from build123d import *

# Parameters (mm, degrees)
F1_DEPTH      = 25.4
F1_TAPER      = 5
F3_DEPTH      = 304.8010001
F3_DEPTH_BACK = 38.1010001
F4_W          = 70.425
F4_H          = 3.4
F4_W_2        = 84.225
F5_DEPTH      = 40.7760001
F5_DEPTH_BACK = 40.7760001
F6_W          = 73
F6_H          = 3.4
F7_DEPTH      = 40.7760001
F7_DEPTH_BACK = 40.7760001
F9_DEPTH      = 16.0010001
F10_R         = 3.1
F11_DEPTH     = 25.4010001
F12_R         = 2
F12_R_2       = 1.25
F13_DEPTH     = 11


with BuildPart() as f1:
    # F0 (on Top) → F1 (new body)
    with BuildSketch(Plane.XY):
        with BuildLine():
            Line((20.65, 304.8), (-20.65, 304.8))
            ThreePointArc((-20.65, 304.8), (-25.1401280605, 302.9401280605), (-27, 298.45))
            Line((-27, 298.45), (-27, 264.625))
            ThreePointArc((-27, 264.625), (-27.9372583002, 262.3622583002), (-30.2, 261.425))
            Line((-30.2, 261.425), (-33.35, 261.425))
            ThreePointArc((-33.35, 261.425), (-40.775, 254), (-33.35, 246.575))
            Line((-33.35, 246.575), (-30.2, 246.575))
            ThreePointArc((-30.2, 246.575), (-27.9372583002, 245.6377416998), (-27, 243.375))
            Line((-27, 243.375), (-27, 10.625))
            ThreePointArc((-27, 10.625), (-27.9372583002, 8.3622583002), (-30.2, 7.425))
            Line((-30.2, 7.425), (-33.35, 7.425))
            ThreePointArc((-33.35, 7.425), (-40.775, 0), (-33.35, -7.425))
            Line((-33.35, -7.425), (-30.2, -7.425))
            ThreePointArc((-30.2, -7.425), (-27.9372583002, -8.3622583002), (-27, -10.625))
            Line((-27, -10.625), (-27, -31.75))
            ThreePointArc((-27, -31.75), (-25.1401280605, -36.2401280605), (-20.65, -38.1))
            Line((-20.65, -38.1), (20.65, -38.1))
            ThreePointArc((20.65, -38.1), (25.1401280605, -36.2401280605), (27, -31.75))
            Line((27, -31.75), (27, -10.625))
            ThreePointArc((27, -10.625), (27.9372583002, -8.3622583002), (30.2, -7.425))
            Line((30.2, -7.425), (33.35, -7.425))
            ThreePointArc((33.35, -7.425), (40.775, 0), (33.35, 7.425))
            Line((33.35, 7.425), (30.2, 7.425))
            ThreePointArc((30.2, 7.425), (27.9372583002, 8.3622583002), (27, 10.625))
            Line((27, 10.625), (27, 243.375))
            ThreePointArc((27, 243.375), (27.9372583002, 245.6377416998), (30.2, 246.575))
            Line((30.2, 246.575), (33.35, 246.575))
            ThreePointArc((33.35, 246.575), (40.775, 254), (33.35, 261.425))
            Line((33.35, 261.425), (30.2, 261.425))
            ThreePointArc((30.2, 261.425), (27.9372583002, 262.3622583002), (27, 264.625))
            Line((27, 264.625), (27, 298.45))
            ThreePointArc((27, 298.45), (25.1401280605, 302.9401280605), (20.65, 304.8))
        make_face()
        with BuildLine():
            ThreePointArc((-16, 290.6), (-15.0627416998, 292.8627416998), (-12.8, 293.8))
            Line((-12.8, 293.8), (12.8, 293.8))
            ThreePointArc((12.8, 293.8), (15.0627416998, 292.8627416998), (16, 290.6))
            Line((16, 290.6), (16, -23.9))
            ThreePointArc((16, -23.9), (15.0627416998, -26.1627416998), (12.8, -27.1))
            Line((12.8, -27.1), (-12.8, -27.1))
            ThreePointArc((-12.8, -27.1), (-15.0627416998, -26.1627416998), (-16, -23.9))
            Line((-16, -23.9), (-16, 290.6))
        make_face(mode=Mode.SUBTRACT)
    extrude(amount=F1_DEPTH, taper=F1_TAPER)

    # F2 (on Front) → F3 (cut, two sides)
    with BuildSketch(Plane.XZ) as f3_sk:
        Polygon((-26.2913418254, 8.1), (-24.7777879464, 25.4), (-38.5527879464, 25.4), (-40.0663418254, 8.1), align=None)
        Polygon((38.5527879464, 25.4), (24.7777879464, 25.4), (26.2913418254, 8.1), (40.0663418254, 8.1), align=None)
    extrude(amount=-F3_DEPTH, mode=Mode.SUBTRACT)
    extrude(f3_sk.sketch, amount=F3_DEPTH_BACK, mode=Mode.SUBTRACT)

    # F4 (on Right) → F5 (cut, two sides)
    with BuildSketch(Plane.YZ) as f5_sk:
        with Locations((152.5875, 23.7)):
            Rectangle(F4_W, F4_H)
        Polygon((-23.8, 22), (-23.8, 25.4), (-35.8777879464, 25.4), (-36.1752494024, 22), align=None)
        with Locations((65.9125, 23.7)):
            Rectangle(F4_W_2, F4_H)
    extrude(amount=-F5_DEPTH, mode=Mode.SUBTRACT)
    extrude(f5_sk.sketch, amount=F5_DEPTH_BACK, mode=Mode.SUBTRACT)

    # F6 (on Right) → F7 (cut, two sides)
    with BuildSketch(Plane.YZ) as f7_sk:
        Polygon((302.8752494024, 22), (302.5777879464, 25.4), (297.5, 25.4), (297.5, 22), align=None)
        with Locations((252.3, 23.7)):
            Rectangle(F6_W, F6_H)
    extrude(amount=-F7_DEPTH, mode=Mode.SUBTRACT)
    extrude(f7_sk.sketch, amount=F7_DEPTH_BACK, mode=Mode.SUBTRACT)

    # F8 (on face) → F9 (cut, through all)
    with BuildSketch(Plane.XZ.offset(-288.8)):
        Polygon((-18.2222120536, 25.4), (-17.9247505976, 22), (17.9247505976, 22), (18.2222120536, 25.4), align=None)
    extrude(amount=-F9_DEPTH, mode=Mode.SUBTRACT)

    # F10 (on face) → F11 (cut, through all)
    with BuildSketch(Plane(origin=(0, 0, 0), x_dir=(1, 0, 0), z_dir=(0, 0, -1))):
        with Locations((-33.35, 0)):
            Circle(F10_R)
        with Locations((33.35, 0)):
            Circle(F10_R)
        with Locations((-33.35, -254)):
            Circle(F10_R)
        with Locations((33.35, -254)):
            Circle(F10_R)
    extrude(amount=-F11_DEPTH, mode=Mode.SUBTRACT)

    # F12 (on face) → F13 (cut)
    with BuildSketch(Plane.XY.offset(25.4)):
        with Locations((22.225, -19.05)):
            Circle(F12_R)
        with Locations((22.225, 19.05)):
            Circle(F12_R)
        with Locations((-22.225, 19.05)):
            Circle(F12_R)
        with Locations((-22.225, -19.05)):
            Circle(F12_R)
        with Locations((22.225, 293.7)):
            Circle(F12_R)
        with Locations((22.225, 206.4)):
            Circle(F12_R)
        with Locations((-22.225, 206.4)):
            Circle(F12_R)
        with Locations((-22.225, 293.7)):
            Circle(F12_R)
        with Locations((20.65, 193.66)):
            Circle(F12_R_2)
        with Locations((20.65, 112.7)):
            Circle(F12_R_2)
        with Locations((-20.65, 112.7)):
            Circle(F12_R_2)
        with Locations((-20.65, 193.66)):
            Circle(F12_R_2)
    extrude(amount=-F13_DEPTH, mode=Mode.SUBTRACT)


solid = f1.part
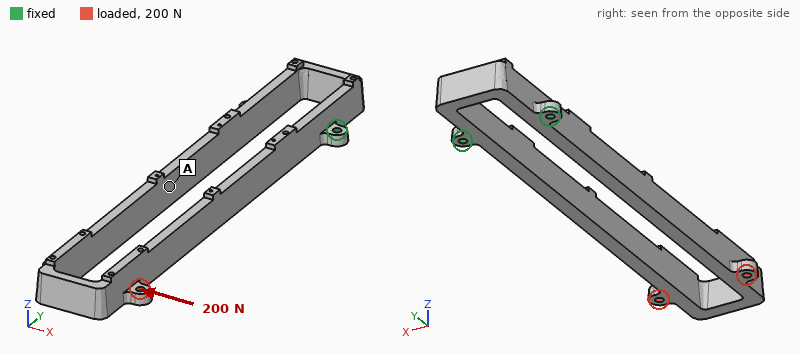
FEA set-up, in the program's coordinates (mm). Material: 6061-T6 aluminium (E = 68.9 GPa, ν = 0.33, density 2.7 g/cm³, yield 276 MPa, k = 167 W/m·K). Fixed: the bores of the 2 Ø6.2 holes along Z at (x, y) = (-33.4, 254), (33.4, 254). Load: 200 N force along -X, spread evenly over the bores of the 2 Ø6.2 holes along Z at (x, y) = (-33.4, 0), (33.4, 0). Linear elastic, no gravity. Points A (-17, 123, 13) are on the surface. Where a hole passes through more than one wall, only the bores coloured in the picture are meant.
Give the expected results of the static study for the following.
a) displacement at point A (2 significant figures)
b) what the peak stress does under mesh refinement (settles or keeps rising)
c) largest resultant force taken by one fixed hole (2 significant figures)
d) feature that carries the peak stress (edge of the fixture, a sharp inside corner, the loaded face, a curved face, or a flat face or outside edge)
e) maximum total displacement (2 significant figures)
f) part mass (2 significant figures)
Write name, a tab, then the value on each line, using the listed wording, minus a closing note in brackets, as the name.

displacement at point A	0.85 mm
what the peak stress does under mesh refinement	keeps rising
largest resultant force taken by one fixed hole	610 N
feature that carries the peak stress	a sharp inside corner
maximum total displacement	1.9 mm
part mass	420 g
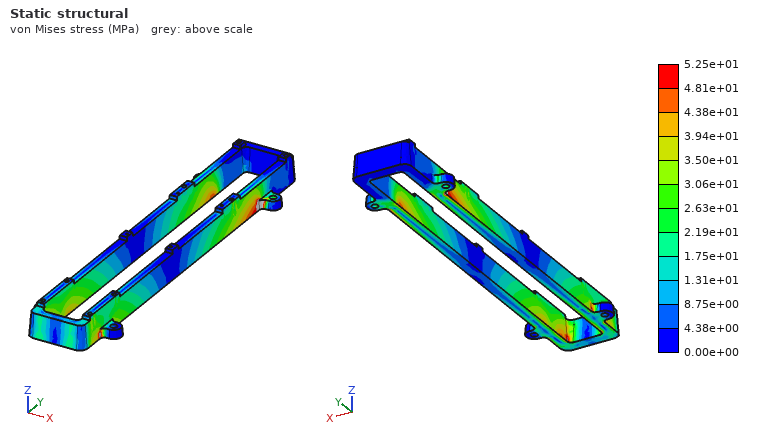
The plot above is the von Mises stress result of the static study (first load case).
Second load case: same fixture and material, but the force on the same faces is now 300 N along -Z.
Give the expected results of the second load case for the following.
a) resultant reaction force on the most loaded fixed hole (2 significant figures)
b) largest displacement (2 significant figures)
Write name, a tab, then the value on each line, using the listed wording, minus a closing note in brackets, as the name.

resultant reaction force on the most loaded fixed hole	160 N
largest displacement	3.3 mm
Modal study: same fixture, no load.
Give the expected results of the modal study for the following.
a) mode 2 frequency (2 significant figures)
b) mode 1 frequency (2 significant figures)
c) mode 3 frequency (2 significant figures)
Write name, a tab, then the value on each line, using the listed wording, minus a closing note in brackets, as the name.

mode 2 frequency	130 Hz
mode 1 frequency	130 Hz
mode 3 frequency	530 Hz
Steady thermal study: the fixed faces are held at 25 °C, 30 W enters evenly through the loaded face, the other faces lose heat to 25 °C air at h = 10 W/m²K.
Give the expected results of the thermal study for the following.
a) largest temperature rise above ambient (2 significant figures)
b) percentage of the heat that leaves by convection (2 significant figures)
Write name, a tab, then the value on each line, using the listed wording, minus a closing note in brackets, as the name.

largest temperature rise above ambient	77 K
percentage of the heat that leaves by convection	55 %
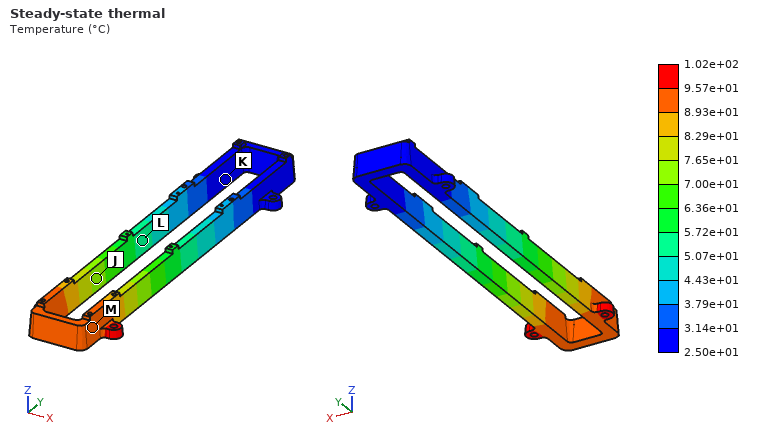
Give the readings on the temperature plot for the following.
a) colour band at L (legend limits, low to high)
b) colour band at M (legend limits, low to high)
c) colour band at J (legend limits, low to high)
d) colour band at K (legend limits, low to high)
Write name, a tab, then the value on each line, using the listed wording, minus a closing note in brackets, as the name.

colour band at L	5.07e+01 to 5.72e+01 °C
colour band at M	8.93e+01 to 9.57e+01 °C
colour band at J	7.00e+01 to 7.65e+01 °C
colour band at K	2.50e+01 to 3.14e+01 °C
